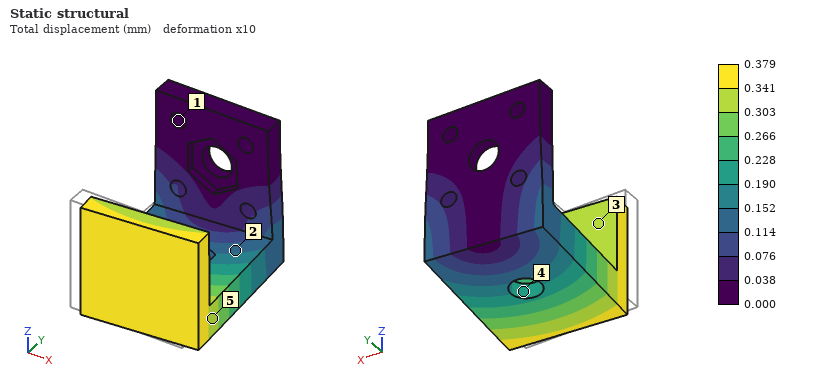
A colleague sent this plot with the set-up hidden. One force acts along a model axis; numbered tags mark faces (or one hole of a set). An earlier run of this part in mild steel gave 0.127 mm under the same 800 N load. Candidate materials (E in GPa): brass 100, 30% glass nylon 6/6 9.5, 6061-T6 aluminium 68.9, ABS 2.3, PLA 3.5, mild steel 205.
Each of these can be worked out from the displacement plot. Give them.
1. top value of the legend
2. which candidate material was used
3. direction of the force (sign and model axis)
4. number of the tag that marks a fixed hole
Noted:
0.379 mm
6061-T6 aluminium
+X
1
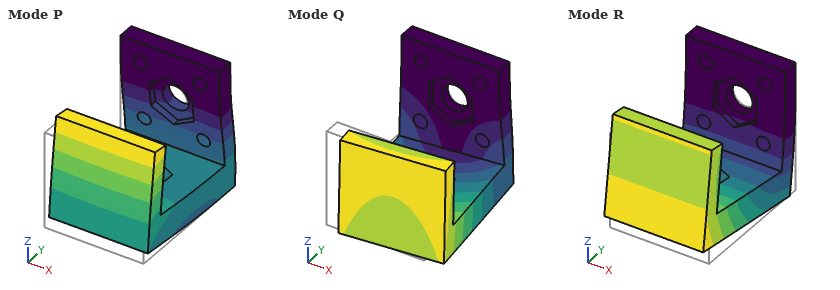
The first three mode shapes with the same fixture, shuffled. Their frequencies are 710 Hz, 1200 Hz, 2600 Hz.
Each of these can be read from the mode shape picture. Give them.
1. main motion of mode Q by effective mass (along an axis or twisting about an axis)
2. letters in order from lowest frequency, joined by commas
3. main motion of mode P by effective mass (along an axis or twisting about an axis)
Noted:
along X
R, Q, P
along Y
